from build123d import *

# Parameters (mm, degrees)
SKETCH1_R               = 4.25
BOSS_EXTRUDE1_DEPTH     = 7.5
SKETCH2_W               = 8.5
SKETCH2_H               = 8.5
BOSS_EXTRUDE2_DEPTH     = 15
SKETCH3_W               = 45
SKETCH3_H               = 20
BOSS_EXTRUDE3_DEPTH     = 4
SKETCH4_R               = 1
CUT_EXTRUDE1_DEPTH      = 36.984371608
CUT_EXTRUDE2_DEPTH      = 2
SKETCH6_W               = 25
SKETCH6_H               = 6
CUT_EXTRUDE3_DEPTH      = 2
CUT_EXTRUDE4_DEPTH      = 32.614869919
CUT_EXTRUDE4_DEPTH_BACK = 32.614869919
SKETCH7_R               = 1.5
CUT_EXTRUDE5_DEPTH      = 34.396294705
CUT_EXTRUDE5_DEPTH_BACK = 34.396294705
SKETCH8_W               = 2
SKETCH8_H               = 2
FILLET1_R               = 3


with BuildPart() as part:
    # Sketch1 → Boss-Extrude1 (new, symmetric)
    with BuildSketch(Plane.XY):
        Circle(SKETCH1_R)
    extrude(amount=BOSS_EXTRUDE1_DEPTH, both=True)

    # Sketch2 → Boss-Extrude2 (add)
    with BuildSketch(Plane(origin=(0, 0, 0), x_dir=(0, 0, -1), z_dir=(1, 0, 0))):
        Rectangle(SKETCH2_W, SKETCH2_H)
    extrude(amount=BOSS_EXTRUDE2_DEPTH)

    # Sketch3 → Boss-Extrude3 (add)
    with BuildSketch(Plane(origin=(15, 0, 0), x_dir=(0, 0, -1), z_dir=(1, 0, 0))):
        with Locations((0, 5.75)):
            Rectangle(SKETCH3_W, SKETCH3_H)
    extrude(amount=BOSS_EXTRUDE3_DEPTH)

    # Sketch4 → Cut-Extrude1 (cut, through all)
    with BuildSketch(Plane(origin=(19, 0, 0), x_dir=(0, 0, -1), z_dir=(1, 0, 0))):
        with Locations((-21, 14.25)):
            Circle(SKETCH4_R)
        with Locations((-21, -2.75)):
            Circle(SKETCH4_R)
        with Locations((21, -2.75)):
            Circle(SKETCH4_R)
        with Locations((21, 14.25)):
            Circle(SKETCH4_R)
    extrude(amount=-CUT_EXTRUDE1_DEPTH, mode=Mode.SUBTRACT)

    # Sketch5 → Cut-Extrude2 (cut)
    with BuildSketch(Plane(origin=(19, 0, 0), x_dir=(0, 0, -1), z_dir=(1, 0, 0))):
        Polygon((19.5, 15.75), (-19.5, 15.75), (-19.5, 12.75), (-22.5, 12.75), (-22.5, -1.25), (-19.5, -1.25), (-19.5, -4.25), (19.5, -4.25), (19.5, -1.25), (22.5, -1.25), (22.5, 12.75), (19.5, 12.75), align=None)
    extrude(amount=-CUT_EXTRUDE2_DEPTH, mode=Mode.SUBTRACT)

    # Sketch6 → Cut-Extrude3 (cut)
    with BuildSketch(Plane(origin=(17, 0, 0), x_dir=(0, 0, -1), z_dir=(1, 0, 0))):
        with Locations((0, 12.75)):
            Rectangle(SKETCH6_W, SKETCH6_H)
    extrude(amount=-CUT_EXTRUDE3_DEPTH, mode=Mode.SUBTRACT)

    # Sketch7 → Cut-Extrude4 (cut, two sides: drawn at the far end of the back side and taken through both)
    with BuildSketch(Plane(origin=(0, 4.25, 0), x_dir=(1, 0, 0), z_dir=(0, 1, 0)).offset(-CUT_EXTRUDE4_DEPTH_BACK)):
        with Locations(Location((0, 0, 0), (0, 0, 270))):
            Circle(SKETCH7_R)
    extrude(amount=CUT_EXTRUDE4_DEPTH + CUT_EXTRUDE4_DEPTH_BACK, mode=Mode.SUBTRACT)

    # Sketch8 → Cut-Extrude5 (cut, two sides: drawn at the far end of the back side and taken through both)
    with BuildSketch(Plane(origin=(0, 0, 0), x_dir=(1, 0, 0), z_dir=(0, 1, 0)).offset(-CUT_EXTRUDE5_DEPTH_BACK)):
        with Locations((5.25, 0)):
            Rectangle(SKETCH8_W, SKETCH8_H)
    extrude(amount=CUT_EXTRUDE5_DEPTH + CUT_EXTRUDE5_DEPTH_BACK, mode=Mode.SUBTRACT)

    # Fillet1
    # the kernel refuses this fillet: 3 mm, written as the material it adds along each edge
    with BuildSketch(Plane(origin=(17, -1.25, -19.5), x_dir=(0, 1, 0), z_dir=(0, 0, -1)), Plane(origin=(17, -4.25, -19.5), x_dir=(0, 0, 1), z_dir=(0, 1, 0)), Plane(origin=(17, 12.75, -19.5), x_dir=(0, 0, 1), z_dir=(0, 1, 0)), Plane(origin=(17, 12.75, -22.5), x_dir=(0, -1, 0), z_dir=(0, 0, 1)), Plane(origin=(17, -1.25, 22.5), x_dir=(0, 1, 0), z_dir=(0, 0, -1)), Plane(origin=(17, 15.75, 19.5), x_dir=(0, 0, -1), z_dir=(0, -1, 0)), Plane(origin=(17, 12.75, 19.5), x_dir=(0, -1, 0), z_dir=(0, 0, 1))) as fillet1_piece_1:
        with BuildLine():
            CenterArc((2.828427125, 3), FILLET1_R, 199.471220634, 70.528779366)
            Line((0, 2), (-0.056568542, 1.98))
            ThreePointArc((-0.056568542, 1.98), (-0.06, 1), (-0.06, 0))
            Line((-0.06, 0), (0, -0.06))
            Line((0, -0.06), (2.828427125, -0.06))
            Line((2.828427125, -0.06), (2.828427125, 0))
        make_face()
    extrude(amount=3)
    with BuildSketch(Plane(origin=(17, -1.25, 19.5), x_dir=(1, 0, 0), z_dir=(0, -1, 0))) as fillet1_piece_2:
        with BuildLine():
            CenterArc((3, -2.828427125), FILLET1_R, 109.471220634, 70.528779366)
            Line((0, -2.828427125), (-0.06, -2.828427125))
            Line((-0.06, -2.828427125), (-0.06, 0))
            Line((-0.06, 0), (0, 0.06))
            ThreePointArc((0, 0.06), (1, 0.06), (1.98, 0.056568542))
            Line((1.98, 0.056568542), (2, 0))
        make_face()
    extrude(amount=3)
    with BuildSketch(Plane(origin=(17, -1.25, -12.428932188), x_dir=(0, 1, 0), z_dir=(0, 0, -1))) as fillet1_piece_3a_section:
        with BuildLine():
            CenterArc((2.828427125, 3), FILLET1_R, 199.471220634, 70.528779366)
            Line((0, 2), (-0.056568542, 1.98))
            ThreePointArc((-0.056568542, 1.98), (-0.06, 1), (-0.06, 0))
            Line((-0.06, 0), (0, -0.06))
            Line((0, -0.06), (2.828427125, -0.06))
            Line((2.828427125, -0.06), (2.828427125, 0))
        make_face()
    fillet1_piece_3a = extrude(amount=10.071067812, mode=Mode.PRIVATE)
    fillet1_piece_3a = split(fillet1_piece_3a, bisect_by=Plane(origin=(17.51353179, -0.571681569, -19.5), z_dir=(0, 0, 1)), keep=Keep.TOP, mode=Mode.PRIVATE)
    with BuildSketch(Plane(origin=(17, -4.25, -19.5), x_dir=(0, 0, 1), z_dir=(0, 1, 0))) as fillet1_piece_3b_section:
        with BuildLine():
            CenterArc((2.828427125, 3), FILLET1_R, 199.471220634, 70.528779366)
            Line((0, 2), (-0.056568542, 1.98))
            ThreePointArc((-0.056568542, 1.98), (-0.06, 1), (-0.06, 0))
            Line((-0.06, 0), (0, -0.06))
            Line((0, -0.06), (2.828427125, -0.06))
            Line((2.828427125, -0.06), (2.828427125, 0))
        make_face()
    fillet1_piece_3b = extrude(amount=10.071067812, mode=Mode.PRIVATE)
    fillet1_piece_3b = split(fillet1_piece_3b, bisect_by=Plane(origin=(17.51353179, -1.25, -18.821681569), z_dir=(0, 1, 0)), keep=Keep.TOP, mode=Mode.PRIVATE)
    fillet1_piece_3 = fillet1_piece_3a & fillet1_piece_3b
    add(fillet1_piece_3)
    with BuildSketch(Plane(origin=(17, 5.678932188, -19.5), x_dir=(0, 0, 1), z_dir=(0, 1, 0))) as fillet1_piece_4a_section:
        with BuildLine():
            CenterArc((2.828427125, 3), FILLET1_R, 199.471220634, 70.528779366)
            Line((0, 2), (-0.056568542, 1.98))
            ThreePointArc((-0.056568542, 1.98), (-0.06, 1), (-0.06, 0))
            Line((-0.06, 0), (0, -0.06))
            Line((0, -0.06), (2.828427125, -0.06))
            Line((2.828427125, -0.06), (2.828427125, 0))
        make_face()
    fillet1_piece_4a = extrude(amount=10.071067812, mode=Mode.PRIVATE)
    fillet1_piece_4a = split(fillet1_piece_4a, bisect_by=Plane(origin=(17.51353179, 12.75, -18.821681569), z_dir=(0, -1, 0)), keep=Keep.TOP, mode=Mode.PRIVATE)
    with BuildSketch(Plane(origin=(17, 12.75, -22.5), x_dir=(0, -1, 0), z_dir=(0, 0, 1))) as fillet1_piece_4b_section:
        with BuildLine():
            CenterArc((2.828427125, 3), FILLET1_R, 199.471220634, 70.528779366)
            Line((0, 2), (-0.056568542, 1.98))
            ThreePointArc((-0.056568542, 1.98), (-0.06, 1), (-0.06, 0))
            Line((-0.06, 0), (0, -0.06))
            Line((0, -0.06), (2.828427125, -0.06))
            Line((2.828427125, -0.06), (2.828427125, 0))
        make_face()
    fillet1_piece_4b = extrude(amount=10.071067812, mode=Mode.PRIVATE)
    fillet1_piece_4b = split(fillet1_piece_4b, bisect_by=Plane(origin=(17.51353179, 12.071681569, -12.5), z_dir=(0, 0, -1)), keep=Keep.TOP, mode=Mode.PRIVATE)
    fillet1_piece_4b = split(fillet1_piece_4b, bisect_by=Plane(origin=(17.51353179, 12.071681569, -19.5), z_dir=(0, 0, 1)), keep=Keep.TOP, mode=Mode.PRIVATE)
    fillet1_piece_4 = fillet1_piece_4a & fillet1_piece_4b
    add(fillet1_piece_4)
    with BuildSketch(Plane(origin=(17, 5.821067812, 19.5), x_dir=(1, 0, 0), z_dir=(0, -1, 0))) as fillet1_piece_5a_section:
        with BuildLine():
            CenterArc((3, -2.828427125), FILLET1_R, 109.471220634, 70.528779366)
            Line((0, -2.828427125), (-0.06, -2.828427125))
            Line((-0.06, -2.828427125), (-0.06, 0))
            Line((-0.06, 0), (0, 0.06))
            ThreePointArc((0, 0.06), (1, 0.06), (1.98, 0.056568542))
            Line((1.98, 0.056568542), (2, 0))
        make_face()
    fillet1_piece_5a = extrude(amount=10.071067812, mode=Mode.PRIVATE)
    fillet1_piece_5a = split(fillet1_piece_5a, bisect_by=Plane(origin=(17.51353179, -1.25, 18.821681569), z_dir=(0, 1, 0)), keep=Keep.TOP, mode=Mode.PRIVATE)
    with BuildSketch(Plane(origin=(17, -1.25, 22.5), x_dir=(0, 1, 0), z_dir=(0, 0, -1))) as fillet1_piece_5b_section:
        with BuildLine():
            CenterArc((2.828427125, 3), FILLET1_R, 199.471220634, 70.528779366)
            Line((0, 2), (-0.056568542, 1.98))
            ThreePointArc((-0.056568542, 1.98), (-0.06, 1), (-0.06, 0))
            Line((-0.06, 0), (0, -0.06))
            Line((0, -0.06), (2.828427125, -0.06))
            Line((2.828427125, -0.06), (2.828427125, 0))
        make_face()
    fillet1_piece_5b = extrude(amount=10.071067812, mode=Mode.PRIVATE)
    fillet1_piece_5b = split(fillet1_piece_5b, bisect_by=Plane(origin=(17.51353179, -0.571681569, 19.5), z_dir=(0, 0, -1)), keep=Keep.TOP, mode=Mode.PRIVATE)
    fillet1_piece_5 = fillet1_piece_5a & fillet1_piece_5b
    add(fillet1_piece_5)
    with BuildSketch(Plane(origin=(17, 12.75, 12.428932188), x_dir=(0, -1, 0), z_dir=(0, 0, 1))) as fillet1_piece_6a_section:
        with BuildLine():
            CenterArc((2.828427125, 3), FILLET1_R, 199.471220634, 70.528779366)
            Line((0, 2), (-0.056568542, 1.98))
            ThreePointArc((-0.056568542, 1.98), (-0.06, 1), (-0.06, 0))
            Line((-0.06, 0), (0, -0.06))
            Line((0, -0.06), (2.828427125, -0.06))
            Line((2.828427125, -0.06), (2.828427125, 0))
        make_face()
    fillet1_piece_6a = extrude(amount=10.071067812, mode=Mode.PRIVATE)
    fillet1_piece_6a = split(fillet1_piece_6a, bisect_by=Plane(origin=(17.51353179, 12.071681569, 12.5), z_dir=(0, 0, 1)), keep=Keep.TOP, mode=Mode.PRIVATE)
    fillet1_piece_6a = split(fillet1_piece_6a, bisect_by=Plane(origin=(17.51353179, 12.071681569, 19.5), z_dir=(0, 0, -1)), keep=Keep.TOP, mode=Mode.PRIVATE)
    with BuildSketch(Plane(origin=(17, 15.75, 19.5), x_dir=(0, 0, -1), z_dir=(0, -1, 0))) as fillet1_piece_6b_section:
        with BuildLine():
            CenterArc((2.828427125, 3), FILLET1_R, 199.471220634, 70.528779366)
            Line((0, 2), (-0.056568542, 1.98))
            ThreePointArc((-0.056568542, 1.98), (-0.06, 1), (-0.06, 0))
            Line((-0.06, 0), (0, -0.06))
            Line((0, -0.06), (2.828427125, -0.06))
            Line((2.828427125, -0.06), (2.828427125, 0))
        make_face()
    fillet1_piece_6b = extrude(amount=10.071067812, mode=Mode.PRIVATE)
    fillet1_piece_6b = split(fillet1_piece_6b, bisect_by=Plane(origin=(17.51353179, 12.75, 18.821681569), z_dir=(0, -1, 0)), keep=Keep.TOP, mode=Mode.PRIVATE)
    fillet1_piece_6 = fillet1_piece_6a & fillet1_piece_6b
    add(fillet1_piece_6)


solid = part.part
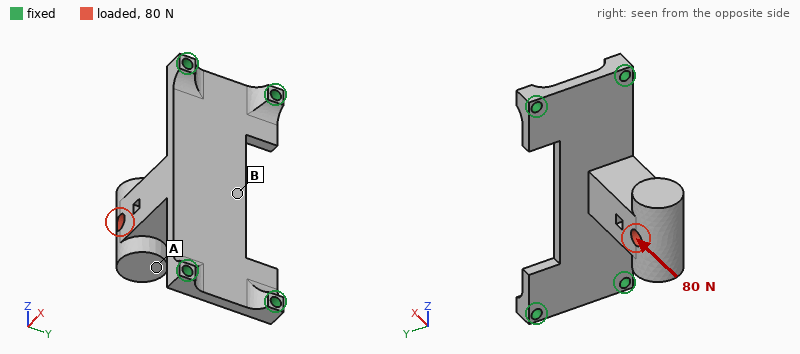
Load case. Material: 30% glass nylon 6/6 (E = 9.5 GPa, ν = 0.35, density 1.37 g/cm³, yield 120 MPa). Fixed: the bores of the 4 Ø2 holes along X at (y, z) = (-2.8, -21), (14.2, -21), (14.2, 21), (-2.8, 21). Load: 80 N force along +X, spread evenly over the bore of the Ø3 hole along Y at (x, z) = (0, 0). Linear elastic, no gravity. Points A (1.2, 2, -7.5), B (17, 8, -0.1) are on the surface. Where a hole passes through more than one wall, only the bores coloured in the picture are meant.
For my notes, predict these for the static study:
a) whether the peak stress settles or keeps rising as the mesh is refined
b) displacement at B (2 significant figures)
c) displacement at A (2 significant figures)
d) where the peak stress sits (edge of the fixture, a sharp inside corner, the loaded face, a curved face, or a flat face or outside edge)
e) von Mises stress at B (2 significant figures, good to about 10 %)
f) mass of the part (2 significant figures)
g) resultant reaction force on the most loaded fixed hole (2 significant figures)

keeps rising
0.14 mm
0.22 mm
edge of the fixture
9.2 MPa
4.3 g
48 N
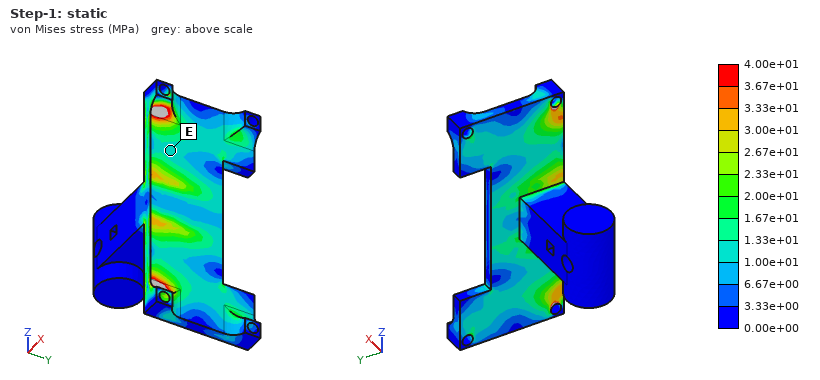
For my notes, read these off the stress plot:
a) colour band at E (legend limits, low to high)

1.00e+01 to 1.33e+01 MPa
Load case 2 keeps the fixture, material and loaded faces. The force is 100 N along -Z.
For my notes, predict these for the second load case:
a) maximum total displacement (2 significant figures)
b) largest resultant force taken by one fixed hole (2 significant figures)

0.56 mm
56 N
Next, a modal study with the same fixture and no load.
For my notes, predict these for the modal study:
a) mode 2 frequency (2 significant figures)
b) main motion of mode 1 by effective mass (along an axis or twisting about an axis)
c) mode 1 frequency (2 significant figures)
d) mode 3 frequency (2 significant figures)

2000 Hz
along Y
1200 Hz
2000 Hz
